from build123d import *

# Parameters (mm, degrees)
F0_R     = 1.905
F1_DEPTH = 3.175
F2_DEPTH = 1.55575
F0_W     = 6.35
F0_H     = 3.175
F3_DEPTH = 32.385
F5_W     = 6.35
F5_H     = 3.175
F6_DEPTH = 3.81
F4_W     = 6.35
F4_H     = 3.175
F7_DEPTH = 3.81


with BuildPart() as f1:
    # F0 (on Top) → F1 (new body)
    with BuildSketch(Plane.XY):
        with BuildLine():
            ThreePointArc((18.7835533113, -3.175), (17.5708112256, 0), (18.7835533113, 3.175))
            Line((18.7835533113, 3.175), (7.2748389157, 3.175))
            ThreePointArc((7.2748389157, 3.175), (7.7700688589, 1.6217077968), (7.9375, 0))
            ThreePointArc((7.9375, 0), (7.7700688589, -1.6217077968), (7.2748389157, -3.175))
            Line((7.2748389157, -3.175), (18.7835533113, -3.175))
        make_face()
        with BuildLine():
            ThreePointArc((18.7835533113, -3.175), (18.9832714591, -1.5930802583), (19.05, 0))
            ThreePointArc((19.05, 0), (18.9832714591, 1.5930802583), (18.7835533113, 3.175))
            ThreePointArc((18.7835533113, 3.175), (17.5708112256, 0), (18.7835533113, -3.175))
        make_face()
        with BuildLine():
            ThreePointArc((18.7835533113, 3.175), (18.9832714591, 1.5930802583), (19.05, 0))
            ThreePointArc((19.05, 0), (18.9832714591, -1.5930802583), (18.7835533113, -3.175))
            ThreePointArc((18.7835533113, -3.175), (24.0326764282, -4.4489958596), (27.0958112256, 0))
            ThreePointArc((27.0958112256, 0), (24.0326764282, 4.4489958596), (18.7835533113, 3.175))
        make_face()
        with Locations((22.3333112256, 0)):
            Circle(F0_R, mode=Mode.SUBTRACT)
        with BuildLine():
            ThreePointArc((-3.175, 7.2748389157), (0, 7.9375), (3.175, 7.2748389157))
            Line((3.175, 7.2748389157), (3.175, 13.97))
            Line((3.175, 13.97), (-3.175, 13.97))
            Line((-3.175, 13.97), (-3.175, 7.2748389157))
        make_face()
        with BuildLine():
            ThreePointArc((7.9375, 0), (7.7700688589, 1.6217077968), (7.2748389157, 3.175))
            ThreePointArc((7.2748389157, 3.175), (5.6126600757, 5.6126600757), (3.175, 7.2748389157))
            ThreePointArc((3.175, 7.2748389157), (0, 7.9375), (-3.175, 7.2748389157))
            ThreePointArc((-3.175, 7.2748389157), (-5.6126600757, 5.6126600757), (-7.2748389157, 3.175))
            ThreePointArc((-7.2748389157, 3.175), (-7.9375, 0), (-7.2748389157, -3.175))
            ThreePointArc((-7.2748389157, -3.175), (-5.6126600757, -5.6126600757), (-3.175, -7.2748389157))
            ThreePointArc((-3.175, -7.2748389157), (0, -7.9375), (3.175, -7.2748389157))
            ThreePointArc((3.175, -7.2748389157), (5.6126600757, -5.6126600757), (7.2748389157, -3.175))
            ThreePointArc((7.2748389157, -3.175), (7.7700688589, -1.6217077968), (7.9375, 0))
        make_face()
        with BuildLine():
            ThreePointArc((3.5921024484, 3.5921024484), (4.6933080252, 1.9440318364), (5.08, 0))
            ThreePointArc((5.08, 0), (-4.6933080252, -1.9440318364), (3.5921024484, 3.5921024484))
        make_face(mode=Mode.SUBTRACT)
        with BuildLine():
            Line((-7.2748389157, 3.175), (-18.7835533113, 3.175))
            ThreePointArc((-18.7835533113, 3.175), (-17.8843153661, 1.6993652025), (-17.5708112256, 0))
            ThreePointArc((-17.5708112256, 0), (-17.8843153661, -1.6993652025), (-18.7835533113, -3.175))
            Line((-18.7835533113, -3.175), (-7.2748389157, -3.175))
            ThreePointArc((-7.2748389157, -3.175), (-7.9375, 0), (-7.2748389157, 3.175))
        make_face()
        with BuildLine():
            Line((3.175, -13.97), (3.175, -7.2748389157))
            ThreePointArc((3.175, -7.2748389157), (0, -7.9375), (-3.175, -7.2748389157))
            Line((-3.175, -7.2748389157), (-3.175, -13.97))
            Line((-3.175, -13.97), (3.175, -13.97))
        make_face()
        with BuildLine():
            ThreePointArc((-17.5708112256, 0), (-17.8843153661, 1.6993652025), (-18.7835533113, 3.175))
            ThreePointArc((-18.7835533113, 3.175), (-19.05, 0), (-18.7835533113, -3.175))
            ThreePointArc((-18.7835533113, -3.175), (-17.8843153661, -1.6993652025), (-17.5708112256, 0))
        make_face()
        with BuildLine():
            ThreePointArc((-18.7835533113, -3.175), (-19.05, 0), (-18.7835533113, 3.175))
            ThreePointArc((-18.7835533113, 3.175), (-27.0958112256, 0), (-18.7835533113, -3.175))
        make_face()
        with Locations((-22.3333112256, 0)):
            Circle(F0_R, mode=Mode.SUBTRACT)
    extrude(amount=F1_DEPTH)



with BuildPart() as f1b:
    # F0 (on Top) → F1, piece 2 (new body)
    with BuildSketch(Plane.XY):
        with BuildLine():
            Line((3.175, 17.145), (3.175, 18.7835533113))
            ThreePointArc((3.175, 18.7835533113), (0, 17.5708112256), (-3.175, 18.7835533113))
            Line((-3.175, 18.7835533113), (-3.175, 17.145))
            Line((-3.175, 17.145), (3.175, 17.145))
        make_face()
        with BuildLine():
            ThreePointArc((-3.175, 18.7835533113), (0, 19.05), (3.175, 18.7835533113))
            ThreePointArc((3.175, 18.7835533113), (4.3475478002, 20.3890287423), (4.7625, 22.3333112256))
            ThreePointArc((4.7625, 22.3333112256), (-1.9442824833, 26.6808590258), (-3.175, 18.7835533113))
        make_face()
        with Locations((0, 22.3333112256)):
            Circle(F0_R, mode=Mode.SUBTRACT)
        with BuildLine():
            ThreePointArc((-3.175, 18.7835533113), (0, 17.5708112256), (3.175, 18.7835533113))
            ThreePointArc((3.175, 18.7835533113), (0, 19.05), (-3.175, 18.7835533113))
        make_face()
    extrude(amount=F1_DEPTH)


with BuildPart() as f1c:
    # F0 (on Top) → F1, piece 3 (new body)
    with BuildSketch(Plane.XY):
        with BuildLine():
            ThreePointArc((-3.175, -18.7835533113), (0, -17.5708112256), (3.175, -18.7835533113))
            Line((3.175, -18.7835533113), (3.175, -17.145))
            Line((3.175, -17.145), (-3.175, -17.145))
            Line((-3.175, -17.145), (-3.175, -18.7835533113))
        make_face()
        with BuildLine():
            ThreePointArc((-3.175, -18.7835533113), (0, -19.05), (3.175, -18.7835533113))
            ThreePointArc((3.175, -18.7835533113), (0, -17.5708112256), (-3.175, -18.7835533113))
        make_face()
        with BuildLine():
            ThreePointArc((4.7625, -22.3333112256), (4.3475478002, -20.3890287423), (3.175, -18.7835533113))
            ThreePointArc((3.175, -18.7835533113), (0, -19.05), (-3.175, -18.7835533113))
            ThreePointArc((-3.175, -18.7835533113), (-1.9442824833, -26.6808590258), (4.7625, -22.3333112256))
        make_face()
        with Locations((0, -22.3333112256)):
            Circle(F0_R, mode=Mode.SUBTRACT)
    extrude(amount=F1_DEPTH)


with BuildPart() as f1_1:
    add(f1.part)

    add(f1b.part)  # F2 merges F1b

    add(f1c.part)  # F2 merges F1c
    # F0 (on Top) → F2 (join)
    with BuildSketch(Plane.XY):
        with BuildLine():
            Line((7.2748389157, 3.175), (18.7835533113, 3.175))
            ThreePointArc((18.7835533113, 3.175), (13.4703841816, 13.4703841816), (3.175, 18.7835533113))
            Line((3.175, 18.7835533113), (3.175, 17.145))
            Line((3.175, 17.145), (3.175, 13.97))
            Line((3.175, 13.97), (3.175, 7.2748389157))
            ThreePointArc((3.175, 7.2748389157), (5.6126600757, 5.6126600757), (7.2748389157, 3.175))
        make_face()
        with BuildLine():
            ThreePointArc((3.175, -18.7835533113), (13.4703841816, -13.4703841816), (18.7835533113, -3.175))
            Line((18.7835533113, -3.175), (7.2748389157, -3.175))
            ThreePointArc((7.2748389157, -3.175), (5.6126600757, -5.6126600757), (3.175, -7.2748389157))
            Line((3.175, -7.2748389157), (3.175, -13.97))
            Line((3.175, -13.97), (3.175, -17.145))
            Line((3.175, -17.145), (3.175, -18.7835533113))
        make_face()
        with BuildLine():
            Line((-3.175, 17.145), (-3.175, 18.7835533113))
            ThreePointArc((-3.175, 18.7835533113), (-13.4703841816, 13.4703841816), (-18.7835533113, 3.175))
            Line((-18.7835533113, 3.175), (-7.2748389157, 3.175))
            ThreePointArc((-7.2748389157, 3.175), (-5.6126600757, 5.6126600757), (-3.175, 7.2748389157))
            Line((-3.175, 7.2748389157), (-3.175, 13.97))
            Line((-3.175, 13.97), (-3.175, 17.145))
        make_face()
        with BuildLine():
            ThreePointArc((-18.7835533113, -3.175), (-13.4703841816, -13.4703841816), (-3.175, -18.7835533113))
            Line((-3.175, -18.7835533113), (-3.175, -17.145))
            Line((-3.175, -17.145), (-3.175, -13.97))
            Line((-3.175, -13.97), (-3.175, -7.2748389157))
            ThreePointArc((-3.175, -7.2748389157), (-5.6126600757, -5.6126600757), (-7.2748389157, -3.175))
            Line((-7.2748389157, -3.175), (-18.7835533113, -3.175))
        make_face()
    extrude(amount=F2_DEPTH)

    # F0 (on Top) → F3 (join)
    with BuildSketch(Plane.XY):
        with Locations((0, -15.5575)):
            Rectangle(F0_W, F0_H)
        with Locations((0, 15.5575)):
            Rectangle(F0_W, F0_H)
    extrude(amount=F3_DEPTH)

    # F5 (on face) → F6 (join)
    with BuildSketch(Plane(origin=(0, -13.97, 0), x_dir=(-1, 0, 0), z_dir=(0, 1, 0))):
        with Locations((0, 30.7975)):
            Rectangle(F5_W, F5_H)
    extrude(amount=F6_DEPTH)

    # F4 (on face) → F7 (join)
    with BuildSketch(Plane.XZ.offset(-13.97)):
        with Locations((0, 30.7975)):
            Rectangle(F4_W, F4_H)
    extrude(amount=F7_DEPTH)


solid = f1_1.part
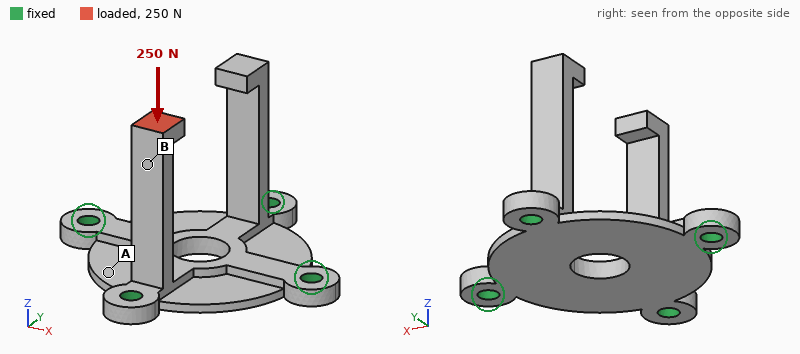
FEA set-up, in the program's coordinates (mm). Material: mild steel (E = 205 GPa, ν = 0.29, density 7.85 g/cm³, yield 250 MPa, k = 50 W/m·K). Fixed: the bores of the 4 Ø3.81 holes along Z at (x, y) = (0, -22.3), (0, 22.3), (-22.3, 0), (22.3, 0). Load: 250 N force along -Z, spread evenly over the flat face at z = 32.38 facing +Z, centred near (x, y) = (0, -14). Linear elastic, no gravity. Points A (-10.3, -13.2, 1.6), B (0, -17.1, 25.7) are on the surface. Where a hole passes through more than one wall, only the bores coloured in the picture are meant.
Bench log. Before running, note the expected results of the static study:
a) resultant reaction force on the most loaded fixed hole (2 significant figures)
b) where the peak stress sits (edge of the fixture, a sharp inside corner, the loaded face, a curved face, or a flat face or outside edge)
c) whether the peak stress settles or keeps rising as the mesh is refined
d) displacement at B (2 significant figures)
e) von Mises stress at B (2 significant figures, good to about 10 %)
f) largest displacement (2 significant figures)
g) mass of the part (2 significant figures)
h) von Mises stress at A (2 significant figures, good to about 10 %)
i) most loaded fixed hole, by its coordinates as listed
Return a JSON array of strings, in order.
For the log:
["210 N", "edge of the fixture", "keeps rising", "52 µm", "31 MPa", "85 µm", "34 g", "9.1 MPa", "(0, -22.3)"]
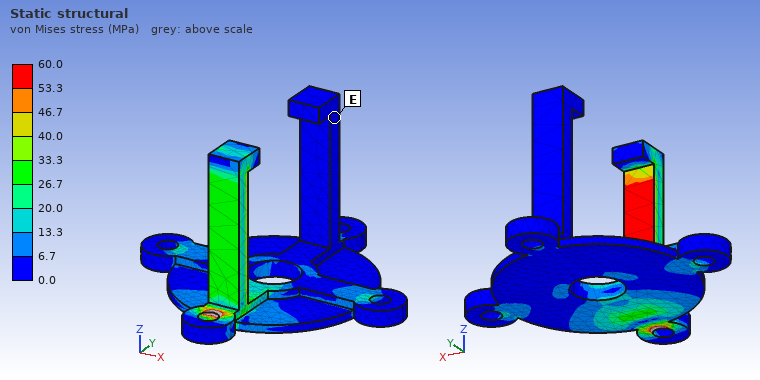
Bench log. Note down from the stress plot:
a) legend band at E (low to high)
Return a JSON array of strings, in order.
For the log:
["0.0 to 6.7 MPa"]
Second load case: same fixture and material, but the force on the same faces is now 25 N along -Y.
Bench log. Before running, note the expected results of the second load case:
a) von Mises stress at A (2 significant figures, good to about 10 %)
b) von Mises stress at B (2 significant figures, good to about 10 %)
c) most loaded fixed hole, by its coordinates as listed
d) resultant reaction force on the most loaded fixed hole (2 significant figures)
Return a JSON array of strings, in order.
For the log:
["5.4 MPa", "15 MPa", "(0, -22.3)", "56 N"]
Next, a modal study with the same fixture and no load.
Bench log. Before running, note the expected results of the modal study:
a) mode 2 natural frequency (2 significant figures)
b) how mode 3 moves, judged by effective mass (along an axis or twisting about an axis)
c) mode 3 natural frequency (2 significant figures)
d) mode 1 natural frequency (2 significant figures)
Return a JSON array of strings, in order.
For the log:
["2200 Hz", "along X", "3300 Hz", "2100 Hz"]
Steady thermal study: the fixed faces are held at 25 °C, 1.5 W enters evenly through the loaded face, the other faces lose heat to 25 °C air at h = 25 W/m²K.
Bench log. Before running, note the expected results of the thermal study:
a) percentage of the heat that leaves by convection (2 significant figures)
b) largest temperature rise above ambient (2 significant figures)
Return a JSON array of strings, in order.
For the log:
["28 %", "41 K"]
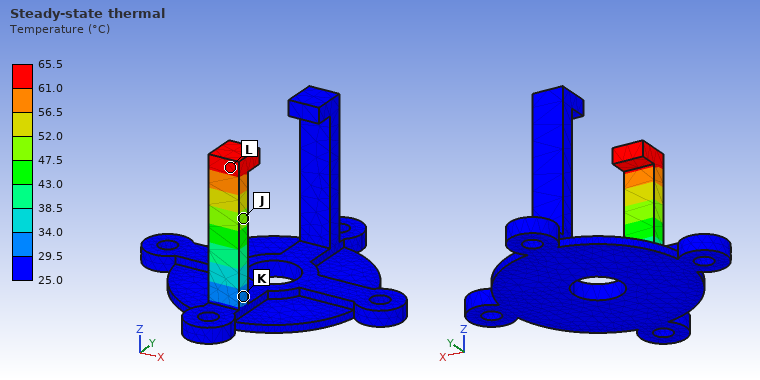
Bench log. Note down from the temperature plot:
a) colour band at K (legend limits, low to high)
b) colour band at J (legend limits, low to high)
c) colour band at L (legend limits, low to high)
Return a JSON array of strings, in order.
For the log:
["29.5 to 34.0 °C", "47.5 to 52.0 °C", "61.0 to 65.5 °C"]
